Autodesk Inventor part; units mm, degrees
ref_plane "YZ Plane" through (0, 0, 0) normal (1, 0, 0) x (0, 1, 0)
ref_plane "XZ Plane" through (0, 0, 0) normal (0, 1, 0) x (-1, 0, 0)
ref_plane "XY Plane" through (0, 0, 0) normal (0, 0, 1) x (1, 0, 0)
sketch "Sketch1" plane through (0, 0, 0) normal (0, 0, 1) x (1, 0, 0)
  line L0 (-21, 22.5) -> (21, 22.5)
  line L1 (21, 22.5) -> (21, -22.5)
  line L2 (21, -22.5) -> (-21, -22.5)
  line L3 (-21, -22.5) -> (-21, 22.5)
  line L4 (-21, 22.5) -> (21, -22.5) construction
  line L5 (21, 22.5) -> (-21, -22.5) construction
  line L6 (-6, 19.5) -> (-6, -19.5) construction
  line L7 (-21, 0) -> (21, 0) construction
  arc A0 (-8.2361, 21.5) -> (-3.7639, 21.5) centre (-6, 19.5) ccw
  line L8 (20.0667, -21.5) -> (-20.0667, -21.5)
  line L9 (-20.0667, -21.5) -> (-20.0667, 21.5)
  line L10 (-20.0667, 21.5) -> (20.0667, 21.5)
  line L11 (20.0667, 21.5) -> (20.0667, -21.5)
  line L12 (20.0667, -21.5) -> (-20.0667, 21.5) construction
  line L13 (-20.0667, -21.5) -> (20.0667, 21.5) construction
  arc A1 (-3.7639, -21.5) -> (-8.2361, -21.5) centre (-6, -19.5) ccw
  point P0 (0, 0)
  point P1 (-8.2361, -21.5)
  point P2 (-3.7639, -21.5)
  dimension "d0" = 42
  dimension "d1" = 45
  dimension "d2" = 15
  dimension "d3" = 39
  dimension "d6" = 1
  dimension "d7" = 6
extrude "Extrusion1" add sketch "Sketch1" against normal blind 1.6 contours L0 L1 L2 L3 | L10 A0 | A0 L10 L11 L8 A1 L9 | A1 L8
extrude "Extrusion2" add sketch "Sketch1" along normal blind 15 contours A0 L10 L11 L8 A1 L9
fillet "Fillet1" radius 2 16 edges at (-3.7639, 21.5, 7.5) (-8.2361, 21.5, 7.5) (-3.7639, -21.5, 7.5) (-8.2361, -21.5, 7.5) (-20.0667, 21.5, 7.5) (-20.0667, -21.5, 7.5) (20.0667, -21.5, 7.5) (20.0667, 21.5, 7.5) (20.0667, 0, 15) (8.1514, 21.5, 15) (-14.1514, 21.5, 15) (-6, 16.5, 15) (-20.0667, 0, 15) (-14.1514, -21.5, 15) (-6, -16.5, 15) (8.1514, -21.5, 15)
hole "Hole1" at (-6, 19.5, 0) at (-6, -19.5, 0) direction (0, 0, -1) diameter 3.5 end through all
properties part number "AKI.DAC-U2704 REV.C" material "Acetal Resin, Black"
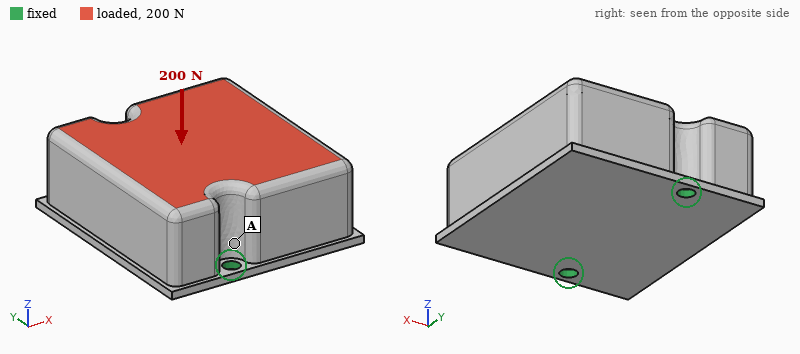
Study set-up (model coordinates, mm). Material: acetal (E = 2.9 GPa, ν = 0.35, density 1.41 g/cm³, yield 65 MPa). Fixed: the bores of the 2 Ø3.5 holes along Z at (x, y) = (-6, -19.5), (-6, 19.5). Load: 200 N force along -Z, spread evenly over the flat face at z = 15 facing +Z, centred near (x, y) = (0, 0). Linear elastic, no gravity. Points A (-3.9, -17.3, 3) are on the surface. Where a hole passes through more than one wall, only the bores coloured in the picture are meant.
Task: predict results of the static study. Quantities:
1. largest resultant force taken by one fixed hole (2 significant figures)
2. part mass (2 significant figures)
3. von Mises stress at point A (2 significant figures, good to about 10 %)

110 N
39 g
7.3 MPa
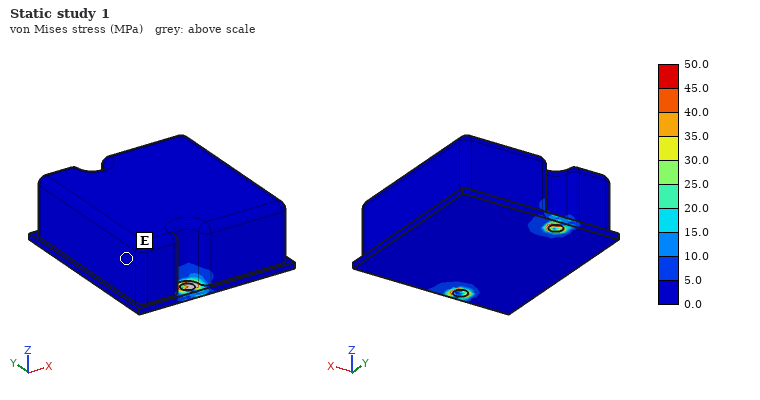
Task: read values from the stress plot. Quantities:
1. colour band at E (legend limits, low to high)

0.0 to 5.0 MPa
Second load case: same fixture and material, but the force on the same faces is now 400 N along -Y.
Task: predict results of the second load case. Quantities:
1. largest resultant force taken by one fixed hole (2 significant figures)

270 N
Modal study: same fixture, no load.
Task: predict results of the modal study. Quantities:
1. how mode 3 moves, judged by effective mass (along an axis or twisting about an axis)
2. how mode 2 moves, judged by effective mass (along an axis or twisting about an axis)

along Y
along Z
